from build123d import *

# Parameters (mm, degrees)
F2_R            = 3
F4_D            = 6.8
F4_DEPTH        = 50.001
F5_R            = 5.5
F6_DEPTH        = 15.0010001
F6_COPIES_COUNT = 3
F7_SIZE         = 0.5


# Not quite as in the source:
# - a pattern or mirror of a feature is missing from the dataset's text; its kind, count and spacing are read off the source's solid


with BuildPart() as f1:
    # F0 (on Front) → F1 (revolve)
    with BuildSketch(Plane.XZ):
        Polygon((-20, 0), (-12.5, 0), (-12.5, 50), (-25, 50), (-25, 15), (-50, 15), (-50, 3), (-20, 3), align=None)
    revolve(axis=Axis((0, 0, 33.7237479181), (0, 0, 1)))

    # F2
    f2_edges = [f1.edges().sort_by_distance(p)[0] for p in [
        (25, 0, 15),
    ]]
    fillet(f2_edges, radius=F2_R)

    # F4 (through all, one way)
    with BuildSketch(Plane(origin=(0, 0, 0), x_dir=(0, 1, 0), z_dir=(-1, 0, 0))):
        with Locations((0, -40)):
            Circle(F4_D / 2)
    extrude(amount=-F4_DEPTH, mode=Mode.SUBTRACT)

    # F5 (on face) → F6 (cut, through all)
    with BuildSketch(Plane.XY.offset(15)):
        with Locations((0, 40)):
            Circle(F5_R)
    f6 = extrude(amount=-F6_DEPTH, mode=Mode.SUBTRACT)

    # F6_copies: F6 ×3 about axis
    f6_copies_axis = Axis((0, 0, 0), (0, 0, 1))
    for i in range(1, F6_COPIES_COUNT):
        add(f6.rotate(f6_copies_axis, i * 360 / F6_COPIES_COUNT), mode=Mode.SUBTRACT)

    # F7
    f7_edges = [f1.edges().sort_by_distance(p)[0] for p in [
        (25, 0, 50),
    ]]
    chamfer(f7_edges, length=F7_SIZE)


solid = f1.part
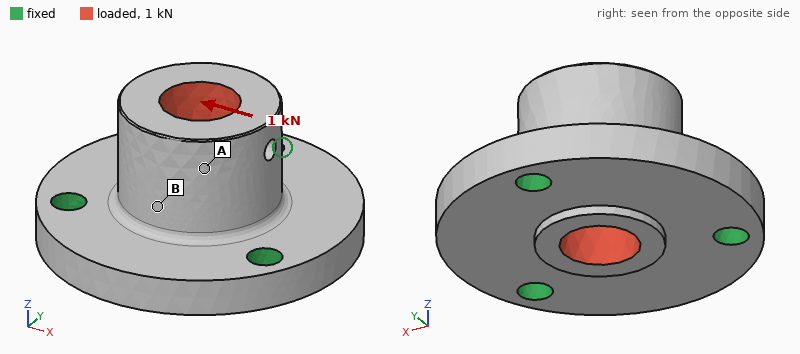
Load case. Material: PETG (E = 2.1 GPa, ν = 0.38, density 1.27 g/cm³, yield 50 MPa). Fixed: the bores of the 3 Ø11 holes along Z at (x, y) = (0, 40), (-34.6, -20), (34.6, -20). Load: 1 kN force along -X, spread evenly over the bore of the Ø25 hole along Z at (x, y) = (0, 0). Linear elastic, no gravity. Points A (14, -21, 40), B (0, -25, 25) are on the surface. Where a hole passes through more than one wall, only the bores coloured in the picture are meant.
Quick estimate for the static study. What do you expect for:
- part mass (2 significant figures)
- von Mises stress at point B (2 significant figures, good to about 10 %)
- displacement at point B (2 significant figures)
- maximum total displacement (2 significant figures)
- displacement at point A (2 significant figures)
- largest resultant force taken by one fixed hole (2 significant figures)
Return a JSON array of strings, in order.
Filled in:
["180 g", "0.80 MPa", "29 µm", "77 µm", "55 µm", "430 N"]
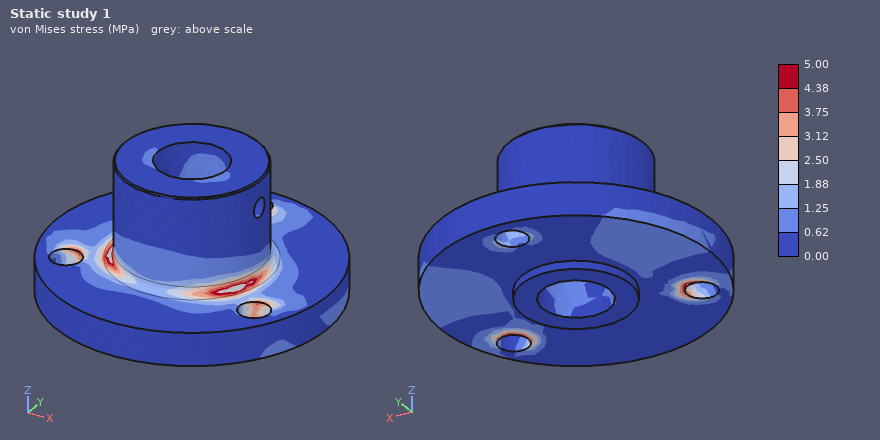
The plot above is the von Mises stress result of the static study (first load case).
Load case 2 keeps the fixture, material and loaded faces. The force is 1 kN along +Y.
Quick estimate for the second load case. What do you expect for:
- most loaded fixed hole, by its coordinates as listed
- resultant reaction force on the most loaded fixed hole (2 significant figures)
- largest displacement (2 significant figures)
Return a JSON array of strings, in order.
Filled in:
["(0, 40)", "470 N", "79 µm"]
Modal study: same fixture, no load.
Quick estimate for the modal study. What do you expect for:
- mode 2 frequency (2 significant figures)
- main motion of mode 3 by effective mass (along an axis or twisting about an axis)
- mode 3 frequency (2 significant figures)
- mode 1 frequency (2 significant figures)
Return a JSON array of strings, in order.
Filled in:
["1900 Hz", "along Z", "2200 Hz", "1900 Hz"]
